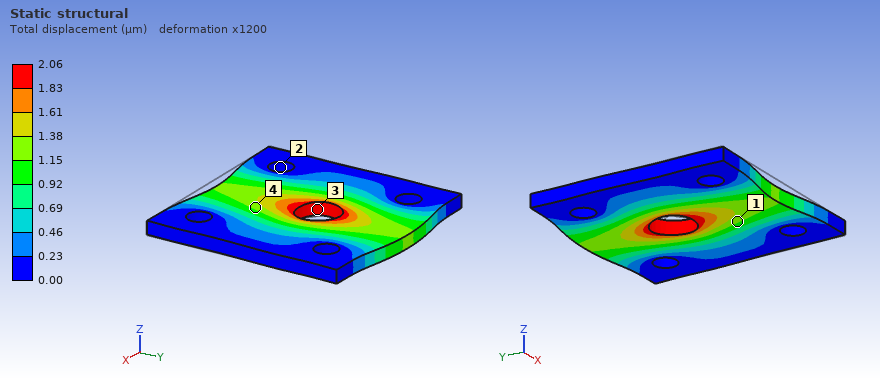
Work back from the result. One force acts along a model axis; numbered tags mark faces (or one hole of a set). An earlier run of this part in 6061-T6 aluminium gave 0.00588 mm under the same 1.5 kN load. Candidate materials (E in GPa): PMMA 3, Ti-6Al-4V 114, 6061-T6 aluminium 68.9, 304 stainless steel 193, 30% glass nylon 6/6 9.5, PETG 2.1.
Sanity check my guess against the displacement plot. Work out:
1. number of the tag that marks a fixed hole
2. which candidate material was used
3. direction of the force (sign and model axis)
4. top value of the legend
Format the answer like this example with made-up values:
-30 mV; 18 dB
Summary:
2; 304 stainless steel; +Y; 2.06 µm
